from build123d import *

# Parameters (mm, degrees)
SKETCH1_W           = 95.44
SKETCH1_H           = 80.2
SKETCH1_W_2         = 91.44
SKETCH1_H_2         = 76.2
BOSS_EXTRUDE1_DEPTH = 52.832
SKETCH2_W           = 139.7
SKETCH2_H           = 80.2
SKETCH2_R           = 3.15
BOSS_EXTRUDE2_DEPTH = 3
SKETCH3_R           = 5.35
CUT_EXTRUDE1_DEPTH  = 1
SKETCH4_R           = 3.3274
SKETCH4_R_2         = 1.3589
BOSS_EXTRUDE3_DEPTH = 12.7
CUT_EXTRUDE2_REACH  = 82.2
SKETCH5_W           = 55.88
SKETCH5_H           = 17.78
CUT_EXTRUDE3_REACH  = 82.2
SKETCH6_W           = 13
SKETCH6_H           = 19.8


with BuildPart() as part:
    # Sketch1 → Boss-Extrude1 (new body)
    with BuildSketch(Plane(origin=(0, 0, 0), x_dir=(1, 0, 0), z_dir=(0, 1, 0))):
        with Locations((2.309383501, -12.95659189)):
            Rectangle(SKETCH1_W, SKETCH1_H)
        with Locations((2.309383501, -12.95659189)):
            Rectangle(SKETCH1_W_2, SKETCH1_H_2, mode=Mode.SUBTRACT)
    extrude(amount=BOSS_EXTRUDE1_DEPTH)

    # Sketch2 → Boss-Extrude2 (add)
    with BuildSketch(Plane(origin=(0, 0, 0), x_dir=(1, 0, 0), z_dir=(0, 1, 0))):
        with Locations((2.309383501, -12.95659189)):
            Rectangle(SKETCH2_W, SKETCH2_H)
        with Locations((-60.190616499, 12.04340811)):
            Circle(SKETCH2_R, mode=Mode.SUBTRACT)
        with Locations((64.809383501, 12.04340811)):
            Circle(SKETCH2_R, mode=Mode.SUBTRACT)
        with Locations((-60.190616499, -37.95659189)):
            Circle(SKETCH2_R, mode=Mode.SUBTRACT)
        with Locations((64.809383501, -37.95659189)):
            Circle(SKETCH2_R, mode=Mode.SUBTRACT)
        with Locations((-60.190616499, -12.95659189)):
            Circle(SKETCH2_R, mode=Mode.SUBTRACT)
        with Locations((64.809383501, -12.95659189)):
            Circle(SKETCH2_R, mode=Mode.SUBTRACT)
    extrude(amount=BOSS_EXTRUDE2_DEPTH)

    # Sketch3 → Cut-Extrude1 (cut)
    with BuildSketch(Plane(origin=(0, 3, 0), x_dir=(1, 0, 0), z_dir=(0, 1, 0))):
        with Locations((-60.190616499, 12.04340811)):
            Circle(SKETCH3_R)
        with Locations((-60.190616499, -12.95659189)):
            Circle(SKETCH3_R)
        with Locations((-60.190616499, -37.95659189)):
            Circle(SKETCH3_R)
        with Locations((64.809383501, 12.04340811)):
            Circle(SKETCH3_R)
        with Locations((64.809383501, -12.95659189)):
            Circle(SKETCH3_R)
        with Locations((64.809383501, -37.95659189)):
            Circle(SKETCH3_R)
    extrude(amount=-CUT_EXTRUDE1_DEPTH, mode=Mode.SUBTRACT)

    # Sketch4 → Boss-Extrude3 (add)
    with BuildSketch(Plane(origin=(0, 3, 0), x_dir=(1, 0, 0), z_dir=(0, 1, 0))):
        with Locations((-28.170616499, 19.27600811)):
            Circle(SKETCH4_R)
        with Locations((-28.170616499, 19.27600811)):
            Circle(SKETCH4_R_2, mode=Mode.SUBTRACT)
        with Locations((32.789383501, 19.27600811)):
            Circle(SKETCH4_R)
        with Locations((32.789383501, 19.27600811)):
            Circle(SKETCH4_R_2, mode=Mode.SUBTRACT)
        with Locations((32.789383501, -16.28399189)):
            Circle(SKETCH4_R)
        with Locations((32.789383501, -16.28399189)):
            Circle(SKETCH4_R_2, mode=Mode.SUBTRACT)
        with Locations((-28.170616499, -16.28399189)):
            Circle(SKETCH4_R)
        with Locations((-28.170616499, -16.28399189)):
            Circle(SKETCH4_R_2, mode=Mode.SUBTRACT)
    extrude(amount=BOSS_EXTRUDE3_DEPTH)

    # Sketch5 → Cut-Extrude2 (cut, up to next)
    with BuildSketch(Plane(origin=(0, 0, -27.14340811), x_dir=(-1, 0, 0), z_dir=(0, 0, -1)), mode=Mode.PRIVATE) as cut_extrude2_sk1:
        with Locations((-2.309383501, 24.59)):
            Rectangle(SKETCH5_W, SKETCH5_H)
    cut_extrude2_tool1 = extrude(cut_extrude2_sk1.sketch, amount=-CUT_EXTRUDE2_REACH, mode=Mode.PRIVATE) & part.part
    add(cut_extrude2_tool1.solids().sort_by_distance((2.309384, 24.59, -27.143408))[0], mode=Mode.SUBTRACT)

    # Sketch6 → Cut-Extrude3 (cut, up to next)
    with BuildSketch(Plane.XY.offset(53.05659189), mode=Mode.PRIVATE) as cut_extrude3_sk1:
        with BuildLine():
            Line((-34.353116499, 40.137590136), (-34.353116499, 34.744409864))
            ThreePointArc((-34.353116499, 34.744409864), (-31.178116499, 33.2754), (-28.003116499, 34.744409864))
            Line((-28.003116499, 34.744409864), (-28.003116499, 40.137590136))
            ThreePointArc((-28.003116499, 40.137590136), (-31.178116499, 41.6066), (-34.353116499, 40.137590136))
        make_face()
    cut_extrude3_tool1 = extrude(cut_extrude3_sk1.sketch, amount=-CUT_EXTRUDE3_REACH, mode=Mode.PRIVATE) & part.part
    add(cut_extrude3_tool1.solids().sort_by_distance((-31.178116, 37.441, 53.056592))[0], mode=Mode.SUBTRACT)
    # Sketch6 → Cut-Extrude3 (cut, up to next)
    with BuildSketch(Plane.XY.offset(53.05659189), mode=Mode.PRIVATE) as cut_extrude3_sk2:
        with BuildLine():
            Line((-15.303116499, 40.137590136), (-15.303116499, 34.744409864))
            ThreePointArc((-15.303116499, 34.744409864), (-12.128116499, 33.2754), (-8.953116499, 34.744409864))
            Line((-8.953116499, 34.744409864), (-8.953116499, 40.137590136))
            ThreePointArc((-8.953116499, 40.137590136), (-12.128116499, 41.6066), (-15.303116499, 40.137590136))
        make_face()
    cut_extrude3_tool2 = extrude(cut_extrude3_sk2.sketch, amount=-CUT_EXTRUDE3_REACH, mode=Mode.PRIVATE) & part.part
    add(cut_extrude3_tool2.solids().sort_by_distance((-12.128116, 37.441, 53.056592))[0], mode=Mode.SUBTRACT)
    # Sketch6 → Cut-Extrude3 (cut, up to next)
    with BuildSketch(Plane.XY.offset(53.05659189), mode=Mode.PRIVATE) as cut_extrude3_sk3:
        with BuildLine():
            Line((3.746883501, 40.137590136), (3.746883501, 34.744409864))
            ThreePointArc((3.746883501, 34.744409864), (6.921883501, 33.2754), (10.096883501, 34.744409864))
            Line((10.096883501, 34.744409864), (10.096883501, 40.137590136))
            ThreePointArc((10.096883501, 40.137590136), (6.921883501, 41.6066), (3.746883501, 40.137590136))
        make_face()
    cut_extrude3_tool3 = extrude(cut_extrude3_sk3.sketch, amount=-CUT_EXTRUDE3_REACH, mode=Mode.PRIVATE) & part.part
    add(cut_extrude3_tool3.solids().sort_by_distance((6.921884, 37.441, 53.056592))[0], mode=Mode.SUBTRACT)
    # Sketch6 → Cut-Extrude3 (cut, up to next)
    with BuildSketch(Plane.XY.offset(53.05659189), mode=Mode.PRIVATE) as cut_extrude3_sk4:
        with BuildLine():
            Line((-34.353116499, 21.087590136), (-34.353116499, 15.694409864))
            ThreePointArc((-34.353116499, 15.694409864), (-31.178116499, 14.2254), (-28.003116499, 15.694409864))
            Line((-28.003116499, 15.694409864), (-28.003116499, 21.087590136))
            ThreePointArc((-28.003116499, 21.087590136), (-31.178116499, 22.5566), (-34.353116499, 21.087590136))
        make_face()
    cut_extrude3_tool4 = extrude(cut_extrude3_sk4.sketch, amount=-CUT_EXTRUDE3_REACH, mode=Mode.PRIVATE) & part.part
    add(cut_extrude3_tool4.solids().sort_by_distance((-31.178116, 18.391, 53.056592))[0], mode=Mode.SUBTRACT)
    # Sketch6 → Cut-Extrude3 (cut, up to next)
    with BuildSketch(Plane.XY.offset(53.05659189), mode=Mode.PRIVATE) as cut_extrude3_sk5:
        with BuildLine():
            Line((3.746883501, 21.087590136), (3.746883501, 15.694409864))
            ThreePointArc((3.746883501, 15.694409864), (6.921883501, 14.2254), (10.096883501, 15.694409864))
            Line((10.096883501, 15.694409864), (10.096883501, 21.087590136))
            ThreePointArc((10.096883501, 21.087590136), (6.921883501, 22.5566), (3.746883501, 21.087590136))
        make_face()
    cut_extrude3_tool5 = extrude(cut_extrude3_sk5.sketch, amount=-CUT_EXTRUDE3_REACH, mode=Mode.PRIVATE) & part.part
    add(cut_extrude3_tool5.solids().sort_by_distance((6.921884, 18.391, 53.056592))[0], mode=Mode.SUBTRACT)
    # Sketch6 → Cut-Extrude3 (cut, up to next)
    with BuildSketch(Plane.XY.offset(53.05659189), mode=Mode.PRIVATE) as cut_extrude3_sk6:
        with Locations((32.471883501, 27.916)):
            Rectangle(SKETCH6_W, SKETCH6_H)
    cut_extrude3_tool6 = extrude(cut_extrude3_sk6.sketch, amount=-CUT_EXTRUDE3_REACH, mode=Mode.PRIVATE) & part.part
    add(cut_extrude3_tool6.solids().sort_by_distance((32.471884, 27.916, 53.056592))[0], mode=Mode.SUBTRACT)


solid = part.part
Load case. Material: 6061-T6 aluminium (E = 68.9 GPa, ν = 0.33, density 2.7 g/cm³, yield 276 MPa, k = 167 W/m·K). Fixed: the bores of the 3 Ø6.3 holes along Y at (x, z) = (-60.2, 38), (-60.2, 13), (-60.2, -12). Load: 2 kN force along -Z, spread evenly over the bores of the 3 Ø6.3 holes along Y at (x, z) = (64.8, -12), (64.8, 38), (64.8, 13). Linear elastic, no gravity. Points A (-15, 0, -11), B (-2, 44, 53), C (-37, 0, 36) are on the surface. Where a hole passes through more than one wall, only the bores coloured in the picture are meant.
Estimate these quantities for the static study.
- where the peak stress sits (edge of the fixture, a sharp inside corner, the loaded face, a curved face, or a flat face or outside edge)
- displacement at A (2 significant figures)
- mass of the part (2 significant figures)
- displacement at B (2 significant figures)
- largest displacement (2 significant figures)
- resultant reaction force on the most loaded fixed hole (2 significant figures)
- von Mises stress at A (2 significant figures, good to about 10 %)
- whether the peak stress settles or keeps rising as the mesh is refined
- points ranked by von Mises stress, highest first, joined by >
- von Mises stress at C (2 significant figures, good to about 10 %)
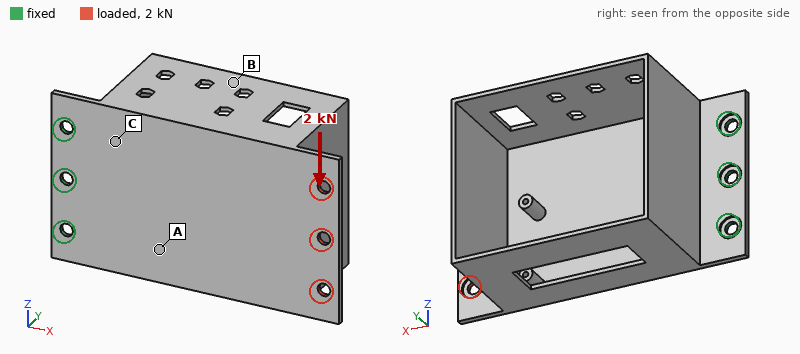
edge of the fixture
0.097 mm
180 g
0.16 mm
0.32 mm
4.7 kN
31 MPa
keeps rising
C > A > B
48 MPa
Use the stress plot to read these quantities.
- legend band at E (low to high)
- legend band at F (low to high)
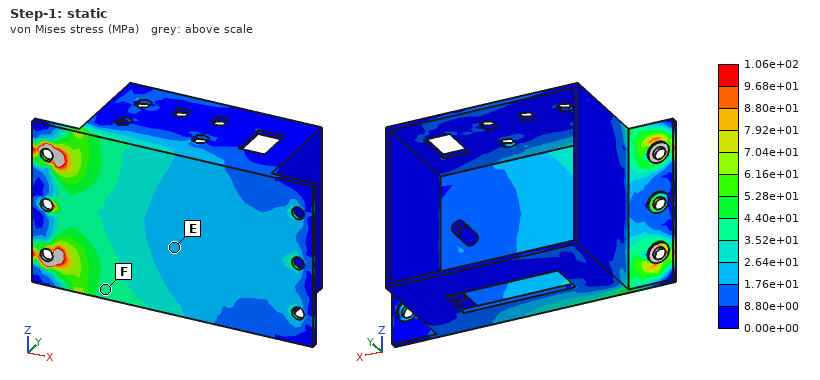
1.76e+01 to 2.64e+01 MPa
3.52e+01 to 4.40e+01 MPa
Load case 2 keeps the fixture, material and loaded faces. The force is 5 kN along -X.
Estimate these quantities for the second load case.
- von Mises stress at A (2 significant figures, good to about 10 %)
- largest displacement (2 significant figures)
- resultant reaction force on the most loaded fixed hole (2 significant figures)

20 MPa
0.54 mm
1.8 kN
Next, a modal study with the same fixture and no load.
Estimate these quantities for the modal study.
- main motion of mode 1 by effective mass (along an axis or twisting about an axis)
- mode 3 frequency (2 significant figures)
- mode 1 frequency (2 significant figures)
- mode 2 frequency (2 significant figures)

along Y
1100 Hz
130 Hz
340 Hz
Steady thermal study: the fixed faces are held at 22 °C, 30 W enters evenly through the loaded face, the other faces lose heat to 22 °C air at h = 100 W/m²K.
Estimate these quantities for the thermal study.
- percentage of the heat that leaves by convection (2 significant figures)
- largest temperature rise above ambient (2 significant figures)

94 %
28 K
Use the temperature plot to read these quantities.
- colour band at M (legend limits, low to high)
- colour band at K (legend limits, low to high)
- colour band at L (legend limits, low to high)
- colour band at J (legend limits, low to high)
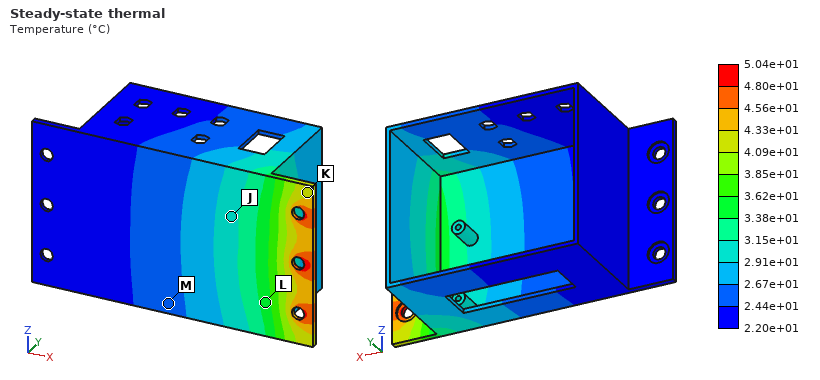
2.44e+01 to 2.67e+01 °C
4.09e+01 to 4.33e+01 °C
3.38e+01 to 3.62e+01 °C
2.91e+01 to 3.15e+01 °C
